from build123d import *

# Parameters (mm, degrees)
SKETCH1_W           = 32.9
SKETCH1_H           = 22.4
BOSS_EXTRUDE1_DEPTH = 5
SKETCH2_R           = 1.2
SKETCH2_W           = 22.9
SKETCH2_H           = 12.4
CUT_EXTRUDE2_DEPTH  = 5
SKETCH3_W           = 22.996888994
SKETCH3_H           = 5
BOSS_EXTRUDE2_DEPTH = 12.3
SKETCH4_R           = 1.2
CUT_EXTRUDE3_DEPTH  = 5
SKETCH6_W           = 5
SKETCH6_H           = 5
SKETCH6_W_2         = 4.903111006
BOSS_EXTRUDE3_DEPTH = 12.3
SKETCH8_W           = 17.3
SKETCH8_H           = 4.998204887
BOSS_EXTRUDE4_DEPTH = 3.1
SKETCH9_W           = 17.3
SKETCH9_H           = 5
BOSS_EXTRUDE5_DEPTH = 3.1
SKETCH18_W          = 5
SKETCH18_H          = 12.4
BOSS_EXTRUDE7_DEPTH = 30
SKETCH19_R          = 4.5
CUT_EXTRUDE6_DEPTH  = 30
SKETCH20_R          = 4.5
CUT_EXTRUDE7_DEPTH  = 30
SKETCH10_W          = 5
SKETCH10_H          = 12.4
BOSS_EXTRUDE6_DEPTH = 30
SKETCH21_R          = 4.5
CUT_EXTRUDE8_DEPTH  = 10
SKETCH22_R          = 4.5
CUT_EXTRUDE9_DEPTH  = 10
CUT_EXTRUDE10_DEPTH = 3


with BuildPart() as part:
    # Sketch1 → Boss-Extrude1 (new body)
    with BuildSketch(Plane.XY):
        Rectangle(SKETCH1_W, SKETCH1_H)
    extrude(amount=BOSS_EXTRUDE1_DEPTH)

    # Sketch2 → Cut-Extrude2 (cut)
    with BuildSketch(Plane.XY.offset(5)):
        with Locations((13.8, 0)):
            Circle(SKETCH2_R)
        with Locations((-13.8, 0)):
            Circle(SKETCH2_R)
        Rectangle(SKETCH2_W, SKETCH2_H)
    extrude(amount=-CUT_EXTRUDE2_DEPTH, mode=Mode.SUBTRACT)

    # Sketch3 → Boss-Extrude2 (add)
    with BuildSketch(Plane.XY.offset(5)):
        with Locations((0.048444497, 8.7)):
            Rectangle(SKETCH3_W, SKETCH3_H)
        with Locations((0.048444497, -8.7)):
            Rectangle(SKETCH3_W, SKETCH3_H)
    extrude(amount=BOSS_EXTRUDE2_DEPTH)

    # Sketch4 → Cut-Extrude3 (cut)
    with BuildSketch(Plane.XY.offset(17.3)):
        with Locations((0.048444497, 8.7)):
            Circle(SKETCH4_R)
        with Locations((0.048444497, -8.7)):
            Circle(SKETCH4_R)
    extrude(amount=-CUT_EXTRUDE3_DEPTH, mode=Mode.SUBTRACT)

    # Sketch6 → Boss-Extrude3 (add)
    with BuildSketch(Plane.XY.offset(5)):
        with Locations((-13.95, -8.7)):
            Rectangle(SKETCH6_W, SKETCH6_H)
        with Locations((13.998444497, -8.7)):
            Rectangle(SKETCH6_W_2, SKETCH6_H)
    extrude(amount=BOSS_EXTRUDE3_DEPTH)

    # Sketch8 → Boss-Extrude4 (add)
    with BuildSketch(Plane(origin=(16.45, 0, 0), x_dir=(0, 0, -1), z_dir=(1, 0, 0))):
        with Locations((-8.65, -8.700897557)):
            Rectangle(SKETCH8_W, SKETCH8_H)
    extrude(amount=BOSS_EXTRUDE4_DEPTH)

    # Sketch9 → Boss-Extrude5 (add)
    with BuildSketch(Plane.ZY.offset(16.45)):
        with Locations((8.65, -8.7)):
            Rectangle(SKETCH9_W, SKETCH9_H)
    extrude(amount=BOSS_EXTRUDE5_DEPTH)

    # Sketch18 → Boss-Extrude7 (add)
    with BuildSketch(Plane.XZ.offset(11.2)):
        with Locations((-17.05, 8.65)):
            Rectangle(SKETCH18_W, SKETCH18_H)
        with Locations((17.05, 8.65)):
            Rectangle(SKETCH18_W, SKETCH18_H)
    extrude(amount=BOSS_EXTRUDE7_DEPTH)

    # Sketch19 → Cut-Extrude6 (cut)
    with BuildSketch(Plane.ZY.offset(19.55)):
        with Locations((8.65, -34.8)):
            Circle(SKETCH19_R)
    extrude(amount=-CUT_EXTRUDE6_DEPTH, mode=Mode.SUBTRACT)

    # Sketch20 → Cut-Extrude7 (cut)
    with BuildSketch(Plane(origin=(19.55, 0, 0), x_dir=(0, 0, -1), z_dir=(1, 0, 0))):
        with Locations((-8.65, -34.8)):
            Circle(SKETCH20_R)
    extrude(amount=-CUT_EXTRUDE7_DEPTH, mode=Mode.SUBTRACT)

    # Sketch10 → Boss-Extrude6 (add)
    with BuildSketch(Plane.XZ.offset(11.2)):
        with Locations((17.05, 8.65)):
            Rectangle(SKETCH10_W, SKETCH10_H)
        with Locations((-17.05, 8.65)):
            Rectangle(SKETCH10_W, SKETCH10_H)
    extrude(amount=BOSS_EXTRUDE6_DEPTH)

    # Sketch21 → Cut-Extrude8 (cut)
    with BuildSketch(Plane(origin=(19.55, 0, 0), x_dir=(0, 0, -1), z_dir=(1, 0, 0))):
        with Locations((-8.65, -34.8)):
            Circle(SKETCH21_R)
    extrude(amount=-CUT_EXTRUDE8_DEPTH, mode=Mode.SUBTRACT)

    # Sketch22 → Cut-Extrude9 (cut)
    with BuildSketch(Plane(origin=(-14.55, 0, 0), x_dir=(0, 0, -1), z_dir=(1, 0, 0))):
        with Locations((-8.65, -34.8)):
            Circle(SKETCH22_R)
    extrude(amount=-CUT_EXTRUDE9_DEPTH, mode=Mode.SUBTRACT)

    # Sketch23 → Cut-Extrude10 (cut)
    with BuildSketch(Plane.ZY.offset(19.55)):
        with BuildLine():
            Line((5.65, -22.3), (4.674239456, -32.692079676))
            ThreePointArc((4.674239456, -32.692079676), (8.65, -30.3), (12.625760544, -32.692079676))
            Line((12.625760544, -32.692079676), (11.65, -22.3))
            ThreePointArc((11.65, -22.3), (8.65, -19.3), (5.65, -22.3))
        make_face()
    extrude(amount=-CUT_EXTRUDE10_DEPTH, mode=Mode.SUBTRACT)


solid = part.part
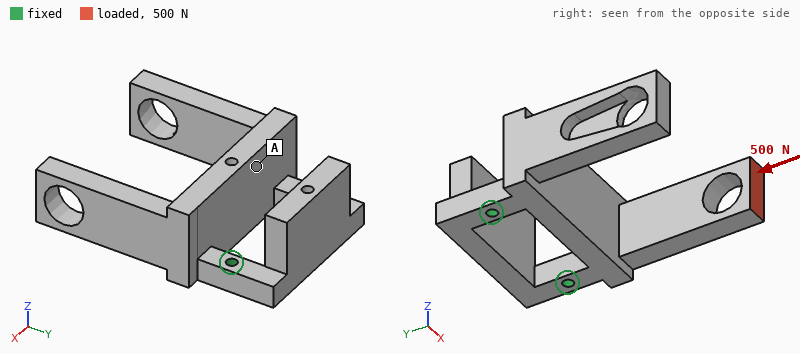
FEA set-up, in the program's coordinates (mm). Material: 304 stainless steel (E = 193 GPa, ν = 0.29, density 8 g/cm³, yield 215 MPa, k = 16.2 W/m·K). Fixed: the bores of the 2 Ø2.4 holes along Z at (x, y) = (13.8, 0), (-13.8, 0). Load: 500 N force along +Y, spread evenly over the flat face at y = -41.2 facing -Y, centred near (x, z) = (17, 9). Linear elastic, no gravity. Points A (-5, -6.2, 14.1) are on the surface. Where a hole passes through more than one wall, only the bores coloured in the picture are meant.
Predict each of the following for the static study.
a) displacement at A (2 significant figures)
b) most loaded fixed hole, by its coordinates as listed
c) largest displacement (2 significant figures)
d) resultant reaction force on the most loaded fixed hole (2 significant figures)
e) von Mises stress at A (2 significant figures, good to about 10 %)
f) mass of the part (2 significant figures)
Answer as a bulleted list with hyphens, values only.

- 11 µm
- (13.8, 0)
- 63 µm
- 550 N
- 13 MPa
- 72 g
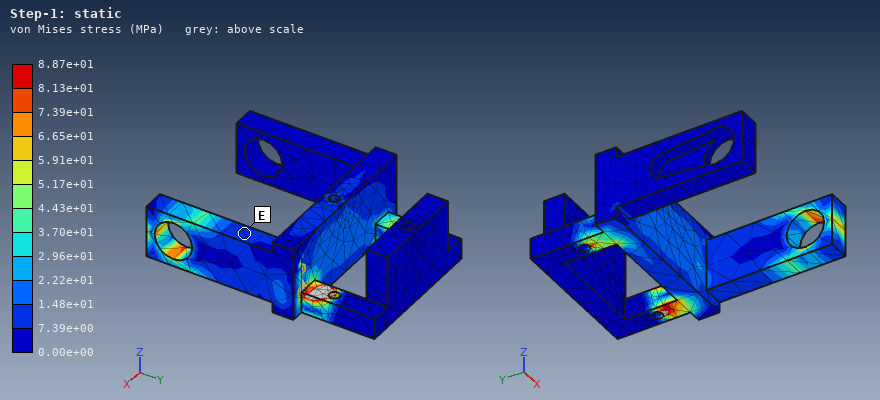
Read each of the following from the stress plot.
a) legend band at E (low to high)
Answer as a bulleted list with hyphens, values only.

- 7.39e+00 to 1.48e+01 MPa
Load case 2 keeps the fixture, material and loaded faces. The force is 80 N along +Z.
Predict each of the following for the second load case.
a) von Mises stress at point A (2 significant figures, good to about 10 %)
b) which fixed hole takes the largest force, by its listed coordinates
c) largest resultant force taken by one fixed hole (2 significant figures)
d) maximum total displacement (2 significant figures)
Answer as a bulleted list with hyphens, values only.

- 12 MPa
- (13.8, 0)
- 82 N
- 70 µm
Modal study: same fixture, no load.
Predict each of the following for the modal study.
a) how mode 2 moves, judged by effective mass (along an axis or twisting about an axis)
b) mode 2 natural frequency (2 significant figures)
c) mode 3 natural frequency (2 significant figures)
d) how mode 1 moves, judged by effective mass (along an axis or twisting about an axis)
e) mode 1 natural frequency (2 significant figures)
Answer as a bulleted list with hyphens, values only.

- along X
- 3300 Hz
- 3600 Hz
- along Z
- 2100 Hz
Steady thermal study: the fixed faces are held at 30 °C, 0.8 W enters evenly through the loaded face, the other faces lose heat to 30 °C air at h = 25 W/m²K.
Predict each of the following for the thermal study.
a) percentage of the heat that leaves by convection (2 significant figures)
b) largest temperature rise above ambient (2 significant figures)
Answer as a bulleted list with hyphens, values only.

- 67 %
- 34 K
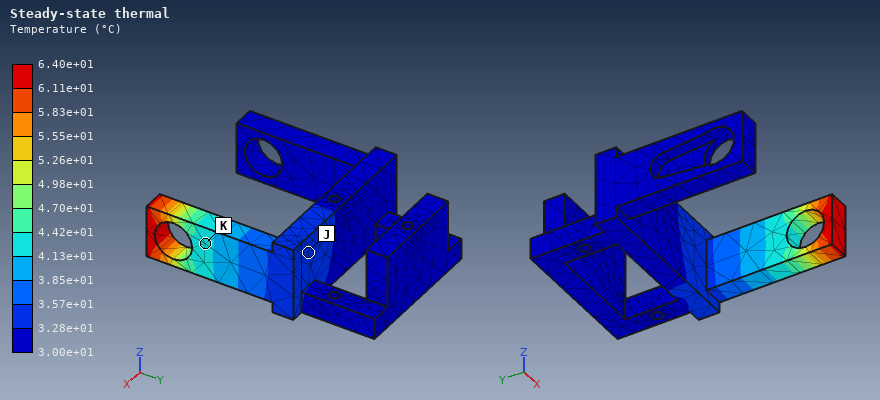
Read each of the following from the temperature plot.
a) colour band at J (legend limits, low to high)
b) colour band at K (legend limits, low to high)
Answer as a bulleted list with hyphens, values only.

- 3.28e+01 to 3.57e+01 °C
- 4.13e+01 to 4.42e+01 °C
